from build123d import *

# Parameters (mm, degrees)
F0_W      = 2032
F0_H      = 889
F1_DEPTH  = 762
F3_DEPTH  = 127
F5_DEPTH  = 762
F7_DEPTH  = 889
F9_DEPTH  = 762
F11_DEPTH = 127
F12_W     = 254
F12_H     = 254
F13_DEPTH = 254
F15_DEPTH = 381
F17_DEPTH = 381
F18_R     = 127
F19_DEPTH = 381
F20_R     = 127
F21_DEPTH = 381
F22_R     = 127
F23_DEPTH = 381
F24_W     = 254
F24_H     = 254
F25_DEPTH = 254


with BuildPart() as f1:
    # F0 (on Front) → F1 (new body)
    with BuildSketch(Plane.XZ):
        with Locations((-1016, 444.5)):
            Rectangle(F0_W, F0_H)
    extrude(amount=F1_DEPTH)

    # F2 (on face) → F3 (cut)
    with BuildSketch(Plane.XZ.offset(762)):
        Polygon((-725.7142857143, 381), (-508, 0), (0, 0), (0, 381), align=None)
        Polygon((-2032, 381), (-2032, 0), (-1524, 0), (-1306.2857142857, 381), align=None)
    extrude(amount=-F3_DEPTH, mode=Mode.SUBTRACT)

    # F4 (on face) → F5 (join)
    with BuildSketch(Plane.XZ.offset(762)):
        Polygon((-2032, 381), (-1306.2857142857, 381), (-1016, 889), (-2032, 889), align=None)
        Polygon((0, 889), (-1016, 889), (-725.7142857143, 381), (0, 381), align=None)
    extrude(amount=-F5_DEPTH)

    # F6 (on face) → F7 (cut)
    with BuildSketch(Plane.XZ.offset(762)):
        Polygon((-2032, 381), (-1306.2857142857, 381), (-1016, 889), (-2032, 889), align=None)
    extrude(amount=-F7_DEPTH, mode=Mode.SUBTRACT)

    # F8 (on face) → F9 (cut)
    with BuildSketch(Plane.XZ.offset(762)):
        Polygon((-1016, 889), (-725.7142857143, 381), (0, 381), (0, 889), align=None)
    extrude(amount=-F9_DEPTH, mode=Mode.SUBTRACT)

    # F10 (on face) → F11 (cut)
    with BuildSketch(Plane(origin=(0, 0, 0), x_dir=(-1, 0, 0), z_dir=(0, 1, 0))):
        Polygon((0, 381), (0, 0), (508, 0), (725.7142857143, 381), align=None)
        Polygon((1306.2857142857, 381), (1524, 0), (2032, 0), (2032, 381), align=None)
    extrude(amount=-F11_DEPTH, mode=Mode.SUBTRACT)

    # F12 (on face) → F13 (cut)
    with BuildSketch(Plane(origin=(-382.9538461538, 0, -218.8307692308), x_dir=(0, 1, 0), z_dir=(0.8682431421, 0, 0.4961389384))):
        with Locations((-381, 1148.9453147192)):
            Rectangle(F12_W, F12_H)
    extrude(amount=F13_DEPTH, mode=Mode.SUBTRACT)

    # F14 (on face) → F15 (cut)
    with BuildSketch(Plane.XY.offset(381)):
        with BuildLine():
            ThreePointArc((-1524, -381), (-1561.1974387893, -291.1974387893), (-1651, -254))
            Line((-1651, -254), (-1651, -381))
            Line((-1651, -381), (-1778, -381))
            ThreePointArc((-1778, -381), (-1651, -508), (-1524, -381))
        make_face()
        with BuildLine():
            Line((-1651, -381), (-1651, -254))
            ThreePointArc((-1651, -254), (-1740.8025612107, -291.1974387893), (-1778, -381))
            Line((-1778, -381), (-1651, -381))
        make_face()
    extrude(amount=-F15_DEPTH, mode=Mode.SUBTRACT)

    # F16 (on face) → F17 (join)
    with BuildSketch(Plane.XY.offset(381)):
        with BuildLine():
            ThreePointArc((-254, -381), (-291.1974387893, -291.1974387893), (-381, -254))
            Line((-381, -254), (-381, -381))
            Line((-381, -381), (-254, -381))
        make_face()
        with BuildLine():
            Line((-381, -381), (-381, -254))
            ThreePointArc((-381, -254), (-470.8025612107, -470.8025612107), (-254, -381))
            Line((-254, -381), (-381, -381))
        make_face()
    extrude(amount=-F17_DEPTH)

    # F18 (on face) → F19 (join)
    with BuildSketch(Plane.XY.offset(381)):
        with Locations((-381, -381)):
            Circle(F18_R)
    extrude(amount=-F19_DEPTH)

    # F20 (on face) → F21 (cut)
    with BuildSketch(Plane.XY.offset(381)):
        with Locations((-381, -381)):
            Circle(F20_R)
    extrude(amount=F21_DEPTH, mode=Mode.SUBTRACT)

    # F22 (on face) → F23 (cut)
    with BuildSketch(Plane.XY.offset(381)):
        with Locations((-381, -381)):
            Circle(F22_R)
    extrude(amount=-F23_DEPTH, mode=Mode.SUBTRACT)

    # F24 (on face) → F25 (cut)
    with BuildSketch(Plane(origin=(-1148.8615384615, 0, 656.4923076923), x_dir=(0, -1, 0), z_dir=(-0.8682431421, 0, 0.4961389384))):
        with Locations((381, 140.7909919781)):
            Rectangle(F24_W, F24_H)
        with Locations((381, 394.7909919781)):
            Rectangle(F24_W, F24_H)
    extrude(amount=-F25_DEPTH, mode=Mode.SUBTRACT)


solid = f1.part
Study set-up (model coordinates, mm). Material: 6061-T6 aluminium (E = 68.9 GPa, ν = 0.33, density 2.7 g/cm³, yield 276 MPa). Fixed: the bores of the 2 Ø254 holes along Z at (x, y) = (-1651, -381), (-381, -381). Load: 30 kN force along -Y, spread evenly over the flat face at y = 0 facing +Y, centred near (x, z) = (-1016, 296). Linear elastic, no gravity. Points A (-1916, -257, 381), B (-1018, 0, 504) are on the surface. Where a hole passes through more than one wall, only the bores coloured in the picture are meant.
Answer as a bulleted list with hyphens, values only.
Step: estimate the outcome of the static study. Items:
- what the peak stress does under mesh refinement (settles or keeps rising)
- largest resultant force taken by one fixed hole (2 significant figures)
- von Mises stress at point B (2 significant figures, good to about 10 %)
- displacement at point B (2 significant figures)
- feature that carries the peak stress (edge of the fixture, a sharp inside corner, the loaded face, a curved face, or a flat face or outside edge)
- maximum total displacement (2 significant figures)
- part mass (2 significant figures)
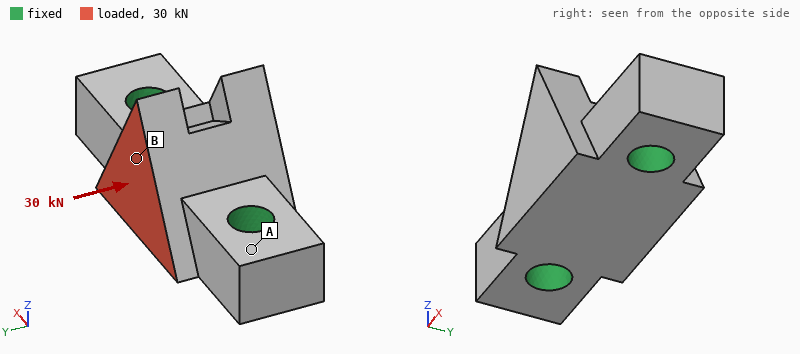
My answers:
- keeps rising
- 15 kN
- 0.12 MPa
- 3.6 µm
- edge of the fixture
- 6.2 µm
- 1400 kg
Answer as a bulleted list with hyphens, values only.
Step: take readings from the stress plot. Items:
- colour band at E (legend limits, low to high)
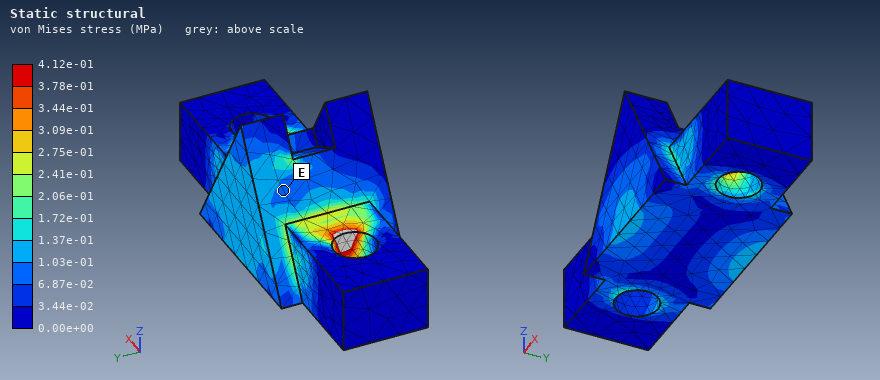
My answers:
- 6.87e-02 to 1.03e-01 MPa
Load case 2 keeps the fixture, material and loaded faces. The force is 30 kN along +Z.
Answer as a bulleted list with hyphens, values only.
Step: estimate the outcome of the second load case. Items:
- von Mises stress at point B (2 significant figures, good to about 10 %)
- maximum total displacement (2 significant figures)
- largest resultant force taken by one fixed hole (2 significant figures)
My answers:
- 0.16 MPa
- 13 µm
- 15 kN
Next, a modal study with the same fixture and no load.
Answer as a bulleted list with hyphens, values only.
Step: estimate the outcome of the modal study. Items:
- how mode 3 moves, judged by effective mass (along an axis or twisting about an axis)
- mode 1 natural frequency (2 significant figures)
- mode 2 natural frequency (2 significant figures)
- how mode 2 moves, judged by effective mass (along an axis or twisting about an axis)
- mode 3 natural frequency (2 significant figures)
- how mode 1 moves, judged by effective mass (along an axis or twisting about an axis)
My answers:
- along Y
- 500 Hz
- 760 Hz
- along Z
- 930 Hz
- along Y
